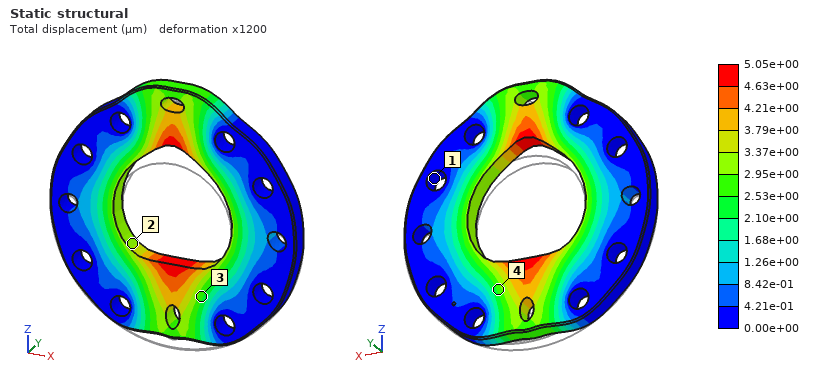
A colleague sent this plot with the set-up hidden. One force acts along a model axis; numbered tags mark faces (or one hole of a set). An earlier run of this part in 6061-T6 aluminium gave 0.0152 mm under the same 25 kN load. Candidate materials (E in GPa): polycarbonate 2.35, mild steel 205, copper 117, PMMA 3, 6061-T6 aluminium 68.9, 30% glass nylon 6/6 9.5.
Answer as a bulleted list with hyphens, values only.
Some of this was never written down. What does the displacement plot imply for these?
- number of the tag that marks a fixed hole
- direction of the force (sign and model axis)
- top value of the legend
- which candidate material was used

- 1
- +Z
- 5.05e+00 µm
- mild steel
